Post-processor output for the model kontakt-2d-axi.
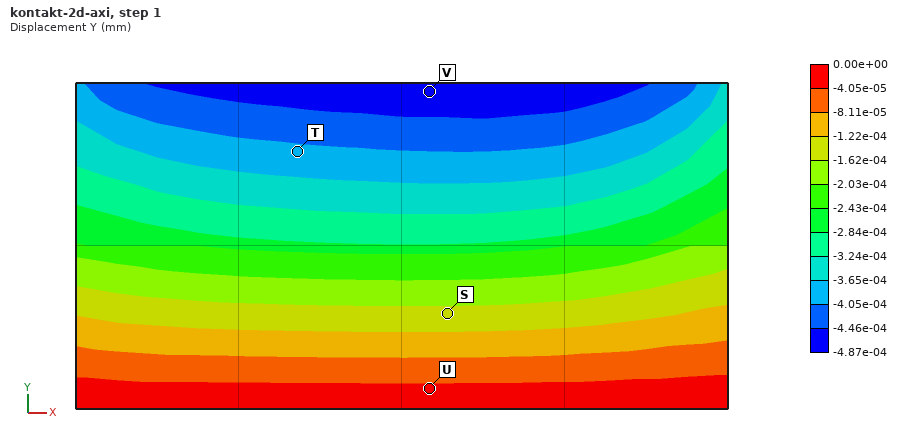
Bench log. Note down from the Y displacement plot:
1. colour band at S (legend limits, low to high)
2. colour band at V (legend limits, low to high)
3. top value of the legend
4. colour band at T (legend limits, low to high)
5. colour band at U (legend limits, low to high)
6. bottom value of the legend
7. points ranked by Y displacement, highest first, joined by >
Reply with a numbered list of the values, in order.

1. -1.62e-04 to -1.22e-04 mm
2. -4.87e-04 to -4.46e-04 mm
3. 0.00e+00 mm
4. -4.05e-04 to -3.65e-04 mm
5. -4.05e-05 to 0.00e+00 mm
6. -4.87e-04 mm
7. U > S > T > V
